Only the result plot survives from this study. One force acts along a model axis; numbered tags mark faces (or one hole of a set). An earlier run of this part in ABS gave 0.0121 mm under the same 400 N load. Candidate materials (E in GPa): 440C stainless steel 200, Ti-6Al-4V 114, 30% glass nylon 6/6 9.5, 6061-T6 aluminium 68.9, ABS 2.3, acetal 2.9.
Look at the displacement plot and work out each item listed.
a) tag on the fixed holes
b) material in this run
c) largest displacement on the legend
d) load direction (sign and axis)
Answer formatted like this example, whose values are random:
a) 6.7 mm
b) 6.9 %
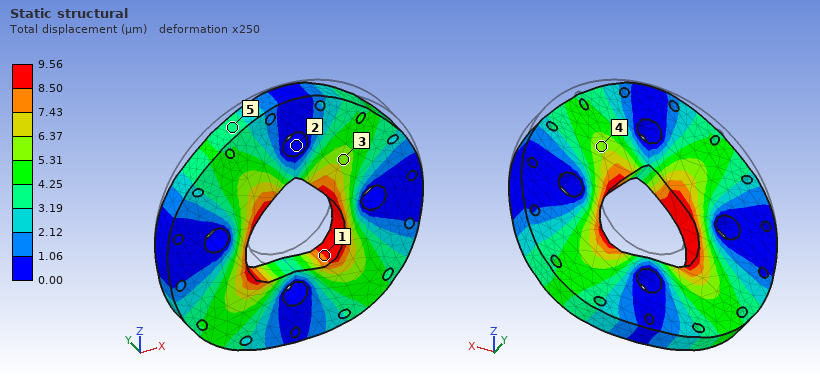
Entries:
a) 2
b) acetal
c) 9.56 µm
d) -Z
